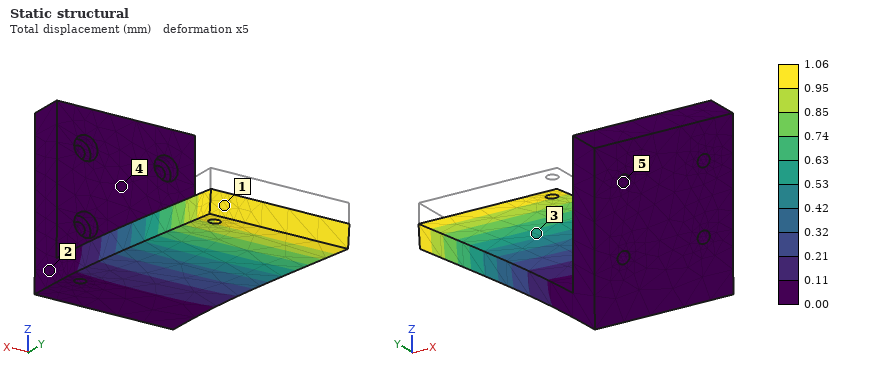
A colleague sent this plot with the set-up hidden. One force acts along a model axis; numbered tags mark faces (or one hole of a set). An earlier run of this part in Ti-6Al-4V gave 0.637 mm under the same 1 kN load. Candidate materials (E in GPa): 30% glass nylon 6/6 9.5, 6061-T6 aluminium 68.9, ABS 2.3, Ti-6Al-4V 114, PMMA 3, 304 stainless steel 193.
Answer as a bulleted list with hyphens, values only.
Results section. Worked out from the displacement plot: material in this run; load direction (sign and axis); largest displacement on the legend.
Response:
- 6061-T6 aluminium
- -Z
- 1.06 mm
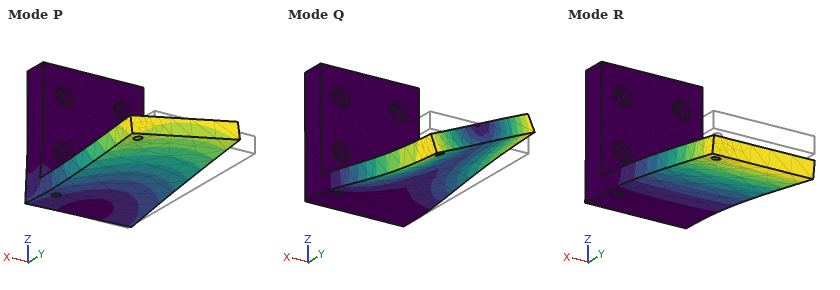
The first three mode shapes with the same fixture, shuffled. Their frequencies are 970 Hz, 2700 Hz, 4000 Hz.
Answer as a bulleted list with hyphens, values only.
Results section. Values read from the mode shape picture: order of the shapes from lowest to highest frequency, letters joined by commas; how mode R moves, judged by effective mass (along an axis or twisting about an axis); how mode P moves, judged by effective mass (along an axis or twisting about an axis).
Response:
- R, P, Q
- along Z
- along X
